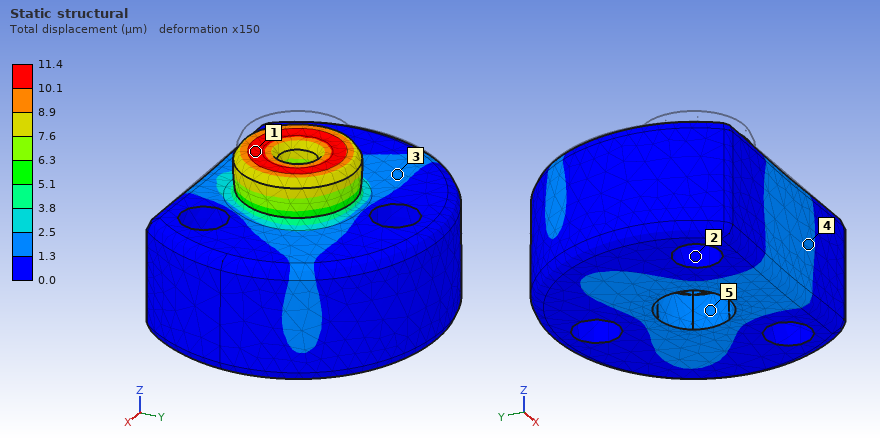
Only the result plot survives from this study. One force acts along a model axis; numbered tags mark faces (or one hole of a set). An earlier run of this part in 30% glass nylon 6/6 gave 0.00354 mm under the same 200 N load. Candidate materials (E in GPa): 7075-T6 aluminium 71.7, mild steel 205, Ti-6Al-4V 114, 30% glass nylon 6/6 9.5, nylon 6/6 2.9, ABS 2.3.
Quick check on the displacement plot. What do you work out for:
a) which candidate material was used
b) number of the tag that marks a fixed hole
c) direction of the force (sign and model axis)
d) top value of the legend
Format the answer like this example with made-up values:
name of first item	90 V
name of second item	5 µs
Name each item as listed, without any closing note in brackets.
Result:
which candidate material was used	nylon 6/6
number of the tag that marks a fixed hole	2
direction of the force	-Z
top value of the legend	11.4 µm
